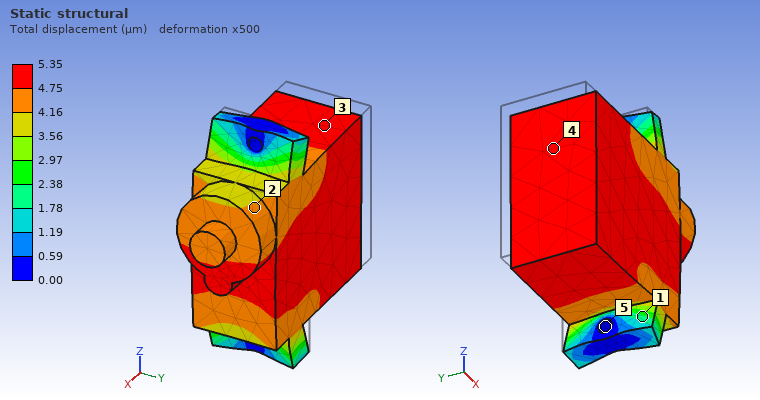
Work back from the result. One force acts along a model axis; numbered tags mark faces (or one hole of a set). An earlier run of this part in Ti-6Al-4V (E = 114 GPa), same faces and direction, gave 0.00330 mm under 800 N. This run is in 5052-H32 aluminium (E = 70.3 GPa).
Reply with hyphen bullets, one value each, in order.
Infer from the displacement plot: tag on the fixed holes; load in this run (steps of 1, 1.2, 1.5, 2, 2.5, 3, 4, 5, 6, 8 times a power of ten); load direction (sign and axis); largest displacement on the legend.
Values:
- 5
- 800 N
- +X
- 5.35 µm
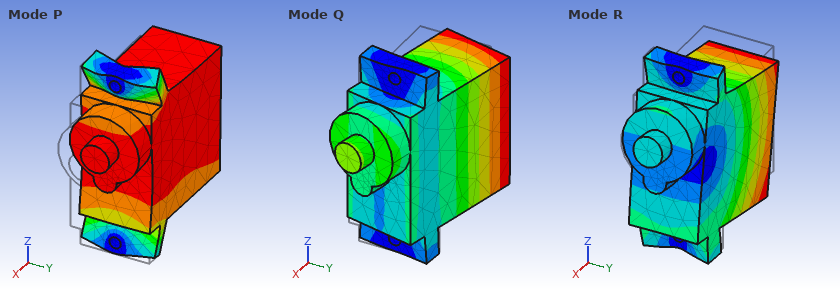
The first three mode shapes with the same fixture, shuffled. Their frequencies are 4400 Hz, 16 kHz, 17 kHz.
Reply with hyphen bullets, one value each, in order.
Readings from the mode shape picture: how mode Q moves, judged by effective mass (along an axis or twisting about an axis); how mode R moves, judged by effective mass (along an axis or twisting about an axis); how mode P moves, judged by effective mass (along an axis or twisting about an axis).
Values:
- along Y
- along Z
- along X
